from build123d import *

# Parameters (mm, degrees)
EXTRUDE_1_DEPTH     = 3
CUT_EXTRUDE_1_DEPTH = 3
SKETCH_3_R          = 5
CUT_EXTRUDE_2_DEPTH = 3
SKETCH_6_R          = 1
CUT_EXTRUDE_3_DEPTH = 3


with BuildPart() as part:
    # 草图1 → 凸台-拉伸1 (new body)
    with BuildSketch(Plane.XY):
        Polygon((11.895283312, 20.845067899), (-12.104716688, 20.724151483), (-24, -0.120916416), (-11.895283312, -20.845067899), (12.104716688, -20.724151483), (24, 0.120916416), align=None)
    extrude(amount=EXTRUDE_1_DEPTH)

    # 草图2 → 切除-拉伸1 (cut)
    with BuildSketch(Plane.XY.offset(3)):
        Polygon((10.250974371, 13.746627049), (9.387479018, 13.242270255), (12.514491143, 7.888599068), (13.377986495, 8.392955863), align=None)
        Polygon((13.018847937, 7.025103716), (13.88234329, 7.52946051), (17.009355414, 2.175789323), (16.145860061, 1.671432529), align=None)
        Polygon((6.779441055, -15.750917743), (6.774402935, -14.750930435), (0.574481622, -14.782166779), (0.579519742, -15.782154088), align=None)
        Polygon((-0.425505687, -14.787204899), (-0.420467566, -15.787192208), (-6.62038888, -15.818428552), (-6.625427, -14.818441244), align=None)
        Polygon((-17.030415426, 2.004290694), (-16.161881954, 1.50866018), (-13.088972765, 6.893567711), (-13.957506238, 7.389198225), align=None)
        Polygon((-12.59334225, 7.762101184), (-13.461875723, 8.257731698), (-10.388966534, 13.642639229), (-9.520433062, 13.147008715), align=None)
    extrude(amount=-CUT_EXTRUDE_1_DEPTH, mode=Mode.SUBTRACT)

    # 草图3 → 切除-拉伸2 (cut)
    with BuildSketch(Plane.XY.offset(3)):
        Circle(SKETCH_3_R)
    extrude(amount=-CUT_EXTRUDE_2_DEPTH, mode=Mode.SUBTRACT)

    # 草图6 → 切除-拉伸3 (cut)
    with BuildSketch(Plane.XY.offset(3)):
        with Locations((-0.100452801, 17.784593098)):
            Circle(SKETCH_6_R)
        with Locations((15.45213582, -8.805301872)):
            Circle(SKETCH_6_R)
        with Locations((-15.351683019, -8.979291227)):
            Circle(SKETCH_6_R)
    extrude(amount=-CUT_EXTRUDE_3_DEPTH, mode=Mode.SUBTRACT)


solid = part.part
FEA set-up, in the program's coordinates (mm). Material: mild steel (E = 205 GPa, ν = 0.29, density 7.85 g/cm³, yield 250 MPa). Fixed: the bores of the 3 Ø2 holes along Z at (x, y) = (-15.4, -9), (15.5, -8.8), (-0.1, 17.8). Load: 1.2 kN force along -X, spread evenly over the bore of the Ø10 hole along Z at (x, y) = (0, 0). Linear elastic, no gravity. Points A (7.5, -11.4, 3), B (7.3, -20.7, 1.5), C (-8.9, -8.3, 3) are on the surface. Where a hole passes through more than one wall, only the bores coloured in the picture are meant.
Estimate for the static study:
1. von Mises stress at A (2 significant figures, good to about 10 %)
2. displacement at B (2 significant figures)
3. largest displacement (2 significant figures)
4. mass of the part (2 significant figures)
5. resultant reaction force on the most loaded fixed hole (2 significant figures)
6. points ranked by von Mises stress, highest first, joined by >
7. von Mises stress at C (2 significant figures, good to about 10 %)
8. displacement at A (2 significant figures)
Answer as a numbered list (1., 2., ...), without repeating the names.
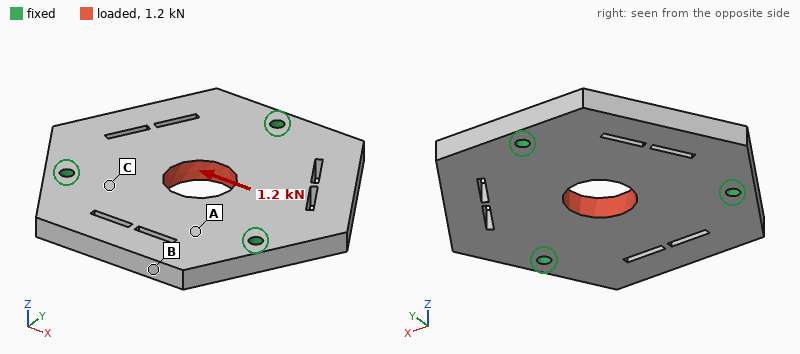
1. 6.8 MPa
2. 0.34 µm
3. 1.6 µm
4. 32 g
5. 410 N
6. C > A > B
7. 13 MPa
8. 0.44 µm
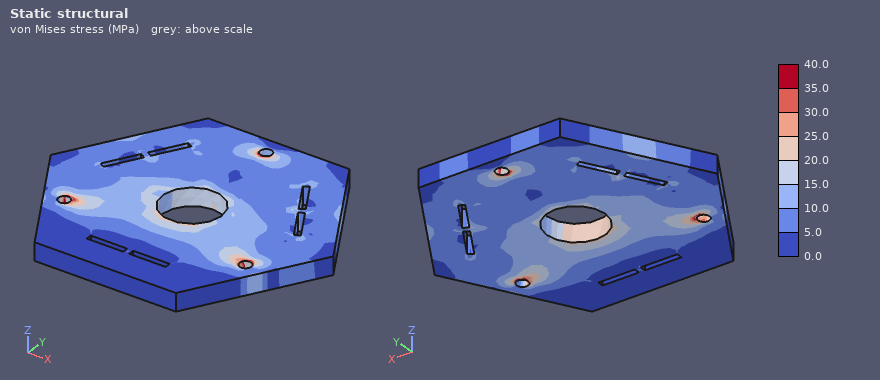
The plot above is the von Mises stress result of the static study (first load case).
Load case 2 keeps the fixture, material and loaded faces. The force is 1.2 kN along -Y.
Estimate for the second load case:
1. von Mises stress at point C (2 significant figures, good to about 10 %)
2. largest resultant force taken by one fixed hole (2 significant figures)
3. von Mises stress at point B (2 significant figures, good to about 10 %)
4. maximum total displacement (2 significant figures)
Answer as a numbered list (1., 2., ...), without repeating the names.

1. 8.8 MPa
2. 410 N
3. 6.2 MPa
4. 1.7 µm
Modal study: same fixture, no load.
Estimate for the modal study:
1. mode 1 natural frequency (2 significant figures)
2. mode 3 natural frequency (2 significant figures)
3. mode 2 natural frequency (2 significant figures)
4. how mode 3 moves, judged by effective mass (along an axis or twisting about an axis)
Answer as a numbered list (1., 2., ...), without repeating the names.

1. 9900 Hz
2. 12 kHz
3. 9900 Hz
4. along Z
